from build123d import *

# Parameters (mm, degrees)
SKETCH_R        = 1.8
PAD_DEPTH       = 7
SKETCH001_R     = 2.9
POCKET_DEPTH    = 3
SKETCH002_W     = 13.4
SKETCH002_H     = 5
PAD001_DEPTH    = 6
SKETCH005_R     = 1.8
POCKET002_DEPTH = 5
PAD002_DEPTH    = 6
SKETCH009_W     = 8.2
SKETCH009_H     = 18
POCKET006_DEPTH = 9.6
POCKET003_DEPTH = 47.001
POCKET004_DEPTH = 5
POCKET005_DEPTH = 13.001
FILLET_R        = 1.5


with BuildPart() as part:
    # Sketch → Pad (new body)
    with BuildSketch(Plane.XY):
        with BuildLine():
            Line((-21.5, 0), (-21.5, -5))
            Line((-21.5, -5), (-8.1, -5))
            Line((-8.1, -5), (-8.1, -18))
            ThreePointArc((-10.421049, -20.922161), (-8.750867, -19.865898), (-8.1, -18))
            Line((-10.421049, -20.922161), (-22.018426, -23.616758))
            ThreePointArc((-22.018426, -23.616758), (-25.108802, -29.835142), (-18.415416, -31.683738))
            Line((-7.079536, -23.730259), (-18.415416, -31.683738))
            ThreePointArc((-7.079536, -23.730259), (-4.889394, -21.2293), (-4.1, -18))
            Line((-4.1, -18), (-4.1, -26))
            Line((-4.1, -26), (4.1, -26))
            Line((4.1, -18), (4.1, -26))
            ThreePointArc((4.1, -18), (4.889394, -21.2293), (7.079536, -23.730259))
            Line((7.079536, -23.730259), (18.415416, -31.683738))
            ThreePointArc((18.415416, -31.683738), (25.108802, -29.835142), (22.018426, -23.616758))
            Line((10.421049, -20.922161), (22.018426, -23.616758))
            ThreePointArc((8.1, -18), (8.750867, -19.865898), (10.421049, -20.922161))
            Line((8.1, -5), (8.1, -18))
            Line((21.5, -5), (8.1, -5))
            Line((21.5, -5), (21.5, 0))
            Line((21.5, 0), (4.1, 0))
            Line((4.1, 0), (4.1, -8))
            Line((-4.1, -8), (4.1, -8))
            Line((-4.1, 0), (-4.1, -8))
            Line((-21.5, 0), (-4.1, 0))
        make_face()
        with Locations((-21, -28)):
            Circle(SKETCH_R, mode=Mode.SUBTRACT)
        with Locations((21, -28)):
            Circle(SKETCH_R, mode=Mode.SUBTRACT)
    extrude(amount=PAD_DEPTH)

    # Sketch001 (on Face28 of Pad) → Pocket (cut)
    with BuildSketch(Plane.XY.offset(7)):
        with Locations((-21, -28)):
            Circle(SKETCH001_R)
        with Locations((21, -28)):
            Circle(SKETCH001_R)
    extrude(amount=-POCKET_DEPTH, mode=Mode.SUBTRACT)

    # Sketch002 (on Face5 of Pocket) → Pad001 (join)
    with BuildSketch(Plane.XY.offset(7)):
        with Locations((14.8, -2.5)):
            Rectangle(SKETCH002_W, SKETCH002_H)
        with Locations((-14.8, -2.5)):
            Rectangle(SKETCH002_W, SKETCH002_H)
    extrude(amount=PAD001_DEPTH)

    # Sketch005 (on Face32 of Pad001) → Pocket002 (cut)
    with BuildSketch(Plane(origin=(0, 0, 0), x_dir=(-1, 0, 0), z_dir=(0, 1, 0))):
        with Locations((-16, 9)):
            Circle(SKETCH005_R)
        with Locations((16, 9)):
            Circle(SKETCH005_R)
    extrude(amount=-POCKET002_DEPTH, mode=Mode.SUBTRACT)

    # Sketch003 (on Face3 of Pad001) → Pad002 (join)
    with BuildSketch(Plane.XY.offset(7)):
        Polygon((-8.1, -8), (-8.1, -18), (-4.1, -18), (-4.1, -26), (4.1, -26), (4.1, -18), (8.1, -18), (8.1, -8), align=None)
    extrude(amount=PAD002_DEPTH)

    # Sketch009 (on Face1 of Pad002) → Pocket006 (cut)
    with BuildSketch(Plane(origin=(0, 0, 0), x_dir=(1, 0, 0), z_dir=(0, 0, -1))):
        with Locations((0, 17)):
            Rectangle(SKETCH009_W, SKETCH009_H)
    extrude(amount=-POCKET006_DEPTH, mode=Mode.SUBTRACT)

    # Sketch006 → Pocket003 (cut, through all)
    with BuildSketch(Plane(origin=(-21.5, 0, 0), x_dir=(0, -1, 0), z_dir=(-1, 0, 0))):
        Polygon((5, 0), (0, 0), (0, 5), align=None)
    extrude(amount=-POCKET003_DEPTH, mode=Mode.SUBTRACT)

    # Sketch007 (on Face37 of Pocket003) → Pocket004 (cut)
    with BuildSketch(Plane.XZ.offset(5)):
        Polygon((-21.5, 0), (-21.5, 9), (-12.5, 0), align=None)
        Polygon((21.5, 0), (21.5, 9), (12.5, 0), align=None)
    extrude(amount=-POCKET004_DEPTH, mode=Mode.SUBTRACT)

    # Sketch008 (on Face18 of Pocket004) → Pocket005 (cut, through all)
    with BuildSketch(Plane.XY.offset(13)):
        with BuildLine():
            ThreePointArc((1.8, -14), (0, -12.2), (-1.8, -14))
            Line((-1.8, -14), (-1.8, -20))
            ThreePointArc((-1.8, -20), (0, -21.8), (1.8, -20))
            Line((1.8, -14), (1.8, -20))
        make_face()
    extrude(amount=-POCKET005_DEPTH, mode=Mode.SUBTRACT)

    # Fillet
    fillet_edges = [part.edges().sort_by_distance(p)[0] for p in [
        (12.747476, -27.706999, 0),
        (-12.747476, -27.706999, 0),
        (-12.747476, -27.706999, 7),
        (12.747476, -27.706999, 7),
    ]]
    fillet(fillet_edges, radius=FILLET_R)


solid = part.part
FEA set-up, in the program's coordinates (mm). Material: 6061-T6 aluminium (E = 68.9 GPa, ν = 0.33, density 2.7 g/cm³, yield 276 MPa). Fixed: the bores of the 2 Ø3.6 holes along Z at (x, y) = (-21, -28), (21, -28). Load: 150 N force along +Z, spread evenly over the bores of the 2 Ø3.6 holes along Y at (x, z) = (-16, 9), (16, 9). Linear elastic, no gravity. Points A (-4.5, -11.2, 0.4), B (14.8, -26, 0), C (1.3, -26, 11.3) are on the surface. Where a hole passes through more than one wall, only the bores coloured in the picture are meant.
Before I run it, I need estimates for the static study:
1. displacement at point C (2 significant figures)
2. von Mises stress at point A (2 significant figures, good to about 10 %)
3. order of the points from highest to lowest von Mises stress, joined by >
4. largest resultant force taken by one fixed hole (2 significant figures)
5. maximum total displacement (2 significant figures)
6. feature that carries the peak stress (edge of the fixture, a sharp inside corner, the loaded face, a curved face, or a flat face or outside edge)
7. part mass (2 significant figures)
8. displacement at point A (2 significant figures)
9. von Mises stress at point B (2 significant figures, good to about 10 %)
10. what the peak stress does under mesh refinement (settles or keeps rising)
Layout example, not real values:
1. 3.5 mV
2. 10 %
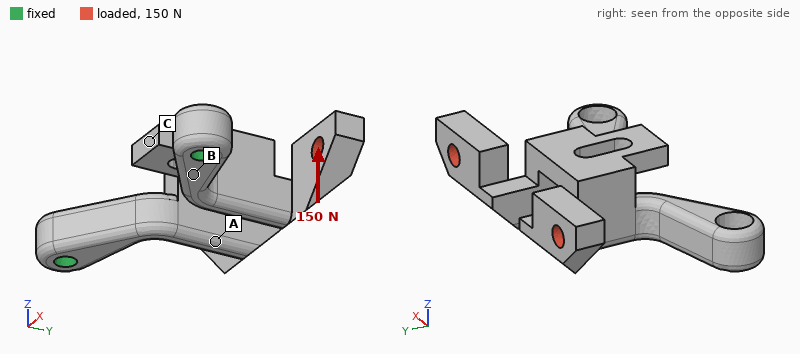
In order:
1. 0.046 mm
2. 21 MPa
3. B > A > C
4. 80 N
5. 0.22 mm
6. edge of the fixture
7. 12 g
8. 0.082 mm
9. 45 MPa
10. keeps rising
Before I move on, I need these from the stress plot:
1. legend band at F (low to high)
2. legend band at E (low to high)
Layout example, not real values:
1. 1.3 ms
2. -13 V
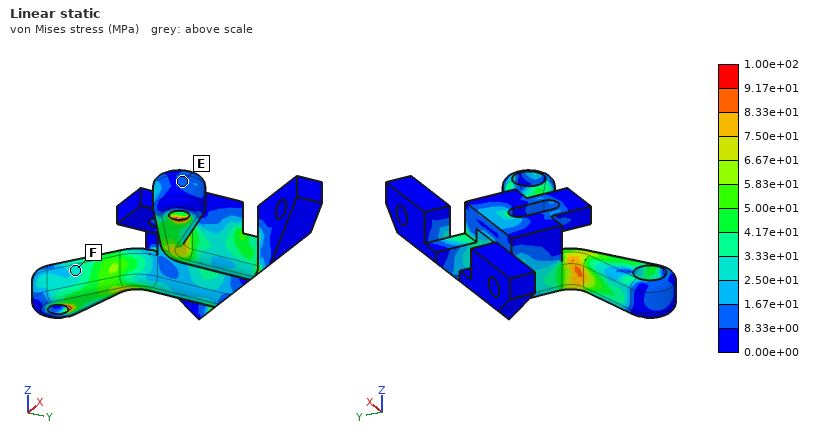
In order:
1. 2.50e+01 to 3.33e+01 MPa
2. 8.33e+00 to 1.67e+01 MPa
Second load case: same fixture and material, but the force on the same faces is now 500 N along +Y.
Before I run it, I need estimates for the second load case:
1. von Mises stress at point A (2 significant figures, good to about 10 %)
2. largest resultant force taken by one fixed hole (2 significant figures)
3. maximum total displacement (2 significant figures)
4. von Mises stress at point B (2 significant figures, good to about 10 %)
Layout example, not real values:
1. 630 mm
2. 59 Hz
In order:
1. 91 MPa
2. 250 N
3. 0.36 mm
4. 23 MPa
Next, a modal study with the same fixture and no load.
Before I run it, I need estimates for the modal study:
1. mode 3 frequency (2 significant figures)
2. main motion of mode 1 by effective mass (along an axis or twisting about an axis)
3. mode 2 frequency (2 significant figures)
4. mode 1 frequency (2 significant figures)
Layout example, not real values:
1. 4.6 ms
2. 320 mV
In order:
1. 4300 Hz
2. along Z
3. 3300 Hz
4. 2300 Hz
